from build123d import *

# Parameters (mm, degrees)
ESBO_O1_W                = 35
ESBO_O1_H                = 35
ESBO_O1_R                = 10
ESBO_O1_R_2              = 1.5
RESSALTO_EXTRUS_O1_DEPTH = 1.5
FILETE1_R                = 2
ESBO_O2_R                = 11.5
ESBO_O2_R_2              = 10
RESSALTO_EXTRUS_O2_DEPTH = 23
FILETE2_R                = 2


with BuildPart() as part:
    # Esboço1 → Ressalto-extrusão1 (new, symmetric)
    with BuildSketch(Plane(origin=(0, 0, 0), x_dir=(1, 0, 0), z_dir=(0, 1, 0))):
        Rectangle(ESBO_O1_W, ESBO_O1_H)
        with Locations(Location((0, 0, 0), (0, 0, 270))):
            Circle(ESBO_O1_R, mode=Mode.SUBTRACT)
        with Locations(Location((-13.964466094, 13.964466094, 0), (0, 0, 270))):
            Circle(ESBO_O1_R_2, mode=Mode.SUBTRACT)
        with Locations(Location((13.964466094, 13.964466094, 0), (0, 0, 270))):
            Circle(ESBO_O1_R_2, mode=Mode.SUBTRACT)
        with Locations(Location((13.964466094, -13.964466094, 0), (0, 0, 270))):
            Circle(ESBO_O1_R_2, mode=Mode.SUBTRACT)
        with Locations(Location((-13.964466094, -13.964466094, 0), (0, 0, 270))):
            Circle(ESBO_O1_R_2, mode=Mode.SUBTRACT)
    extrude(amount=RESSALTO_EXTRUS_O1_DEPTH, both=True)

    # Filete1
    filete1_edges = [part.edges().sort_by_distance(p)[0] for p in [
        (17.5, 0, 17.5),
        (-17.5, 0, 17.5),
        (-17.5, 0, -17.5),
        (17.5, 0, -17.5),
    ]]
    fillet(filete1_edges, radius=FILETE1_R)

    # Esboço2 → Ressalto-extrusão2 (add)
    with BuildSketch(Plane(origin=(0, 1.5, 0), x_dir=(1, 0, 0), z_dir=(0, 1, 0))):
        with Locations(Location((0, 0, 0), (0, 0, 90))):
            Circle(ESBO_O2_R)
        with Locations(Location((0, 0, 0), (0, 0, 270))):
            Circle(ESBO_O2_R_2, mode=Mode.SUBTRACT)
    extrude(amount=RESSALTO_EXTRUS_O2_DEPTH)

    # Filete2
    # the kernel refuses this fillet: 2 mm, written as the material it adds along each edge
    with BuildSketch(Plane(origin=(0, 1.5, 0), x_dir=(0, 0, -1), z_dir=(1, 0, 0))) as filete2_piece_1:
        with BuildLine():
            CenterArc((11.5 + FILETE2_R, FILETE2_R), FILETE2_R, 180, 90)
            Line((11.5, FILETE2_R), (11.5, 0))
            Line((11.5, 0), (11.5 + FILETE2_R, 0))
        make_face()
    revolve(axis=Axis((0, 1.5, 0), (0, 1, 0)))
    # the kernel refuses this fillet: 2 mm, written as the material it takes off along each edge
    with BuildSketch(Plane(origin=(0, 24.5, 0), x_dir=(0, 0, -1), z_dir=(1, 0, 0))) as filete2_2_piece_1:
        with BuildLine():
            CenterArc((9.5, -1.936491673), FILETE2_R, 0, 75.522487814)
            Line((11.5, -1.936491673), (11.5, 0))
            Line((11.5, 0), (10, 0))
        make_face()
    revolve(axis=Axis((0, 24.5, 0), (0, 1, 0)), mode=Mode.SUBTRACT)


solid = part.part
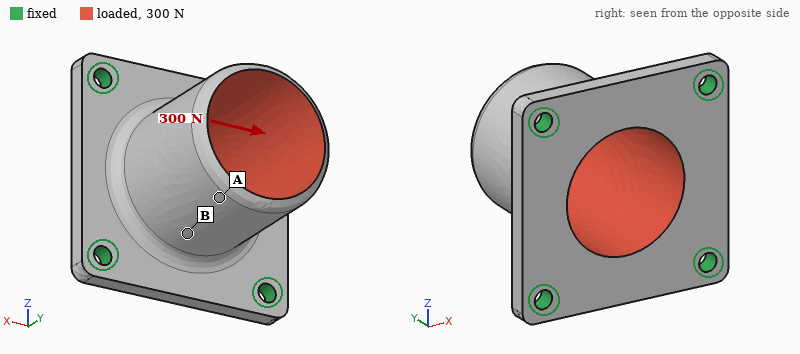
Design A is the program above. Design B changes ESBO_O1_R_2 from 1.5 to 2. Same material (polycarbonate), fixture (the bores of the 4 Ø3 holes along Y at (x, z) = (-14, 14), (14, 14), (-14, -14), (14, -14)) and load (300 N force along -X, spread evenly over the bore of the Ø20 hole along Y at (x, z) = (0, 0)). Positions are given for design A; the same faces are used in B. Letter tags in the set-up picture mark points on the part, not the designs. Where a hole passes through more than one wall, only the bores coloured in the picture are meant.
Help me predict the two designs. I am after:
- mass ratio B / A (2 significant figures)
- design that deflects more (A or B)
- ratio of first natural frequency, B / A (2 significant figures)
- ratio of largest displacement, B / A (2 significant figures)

0.99
A
1.1
0.90
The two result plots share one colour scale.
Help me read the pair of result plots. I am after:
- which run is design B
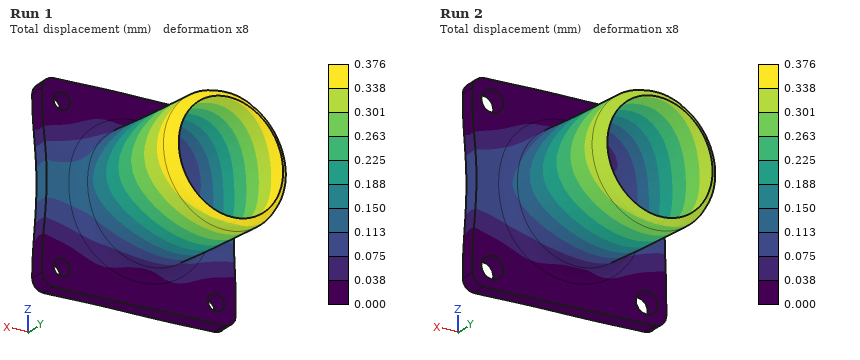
Run 2
